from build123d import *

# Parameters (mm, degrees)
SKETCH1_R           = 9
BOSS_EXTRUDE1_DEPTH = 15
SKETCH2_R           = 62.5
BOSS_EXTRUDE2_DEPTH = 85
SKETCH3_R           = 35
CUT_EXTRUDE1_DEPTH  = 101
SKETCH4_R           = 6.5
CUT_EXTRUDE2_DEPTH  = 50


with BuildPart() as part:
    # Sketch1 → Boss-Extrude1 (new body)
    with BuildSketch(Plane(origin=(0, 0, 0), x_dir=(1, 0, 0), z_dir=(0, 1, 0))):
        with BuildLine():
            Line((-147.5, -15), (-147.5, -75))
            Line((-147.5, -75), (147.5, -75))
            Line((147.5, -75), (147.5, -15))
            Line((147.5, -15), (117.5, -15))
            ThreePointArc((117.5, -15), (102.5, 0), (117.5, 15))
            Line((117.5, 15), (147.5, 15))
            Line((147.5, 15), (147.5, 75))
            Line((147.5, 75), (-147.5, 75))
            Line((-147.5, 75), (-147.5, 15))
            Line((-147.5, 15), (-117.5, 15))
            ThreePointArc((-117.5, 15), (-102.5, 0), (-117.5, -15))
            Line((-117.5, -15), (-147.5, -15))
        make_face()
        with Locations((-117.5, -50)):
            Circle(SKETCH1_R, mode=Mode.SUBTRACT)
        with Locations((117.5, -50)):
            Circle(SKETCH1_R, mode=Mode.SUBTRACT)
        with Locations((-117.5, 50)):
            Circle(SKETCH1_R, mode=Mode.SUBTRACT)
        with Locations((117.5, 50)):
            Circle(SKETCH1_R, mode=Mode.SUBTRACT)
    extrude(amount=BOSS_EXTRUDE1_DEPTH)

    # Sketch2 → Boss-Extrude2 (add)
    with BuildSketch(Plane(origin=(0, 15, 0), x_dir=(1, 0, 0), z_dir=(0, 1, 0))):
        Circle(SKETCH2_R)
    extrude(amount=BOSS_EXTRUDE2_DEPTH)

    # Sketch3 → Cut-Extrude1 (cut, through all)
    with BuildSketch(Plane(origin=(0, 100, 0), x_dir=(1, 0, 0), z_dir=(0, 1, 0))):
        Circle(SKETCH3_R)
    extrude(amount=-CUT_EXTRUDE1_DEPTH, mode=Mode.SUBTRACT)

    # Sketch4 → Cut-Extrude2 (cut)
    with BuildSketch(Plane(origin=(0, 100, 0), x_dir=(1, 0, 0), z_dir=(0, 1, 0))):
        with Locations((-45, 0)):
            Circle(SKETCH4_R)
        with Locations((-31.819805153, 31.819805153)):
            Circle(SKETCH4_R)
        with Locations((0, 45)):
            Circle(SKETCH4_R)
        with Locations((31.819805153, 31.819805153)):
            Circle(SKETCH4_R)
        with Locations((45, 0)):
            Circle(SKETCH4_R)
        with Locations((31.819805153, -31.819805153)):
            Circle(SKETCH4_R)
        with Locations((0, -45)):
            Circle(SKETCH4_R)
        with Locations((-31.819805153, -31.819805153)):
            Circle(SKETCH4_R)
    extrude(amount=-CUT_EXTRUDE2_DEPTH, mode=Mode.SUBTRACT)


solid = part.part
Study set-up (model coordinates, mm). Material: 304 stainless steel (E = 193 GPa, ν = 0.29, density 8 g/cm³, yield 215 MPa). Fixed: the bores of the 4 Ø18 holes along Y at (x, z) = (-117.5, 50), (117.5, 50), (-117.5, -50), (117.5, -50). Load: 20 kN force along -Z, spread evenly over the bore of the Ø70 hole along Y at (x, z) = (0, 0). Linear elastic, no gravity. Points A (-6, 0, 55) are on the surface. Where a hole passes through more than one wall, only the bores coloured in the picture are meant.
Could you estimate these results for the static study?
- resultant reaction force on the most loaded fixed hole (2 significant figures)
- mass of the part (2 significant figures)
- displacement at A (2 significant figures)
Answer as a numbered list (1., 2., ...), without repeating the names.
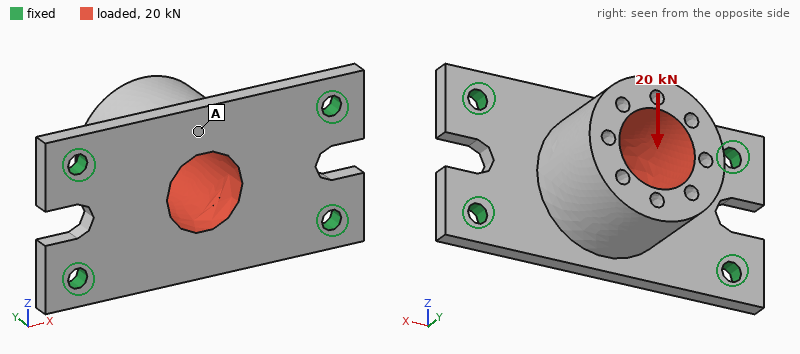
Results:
1. 8.1 kN
2. 9.7 kg
3. 0.047 mm
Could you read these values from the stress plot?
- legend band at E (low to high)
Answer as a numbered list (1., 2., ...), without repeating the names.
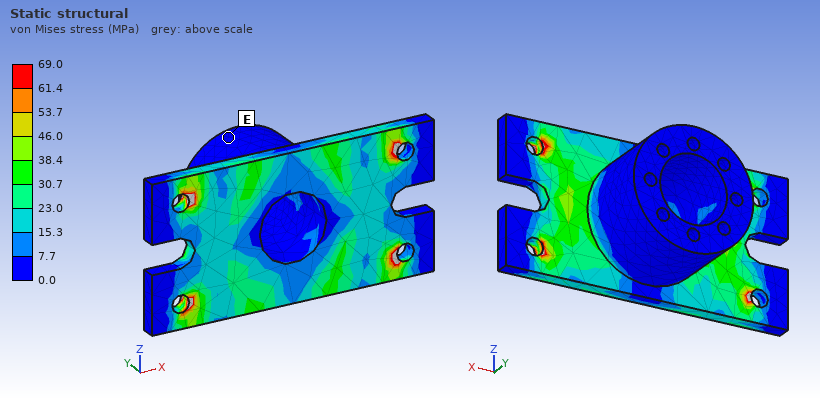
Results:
1. 0.0 to 7.7 MPa
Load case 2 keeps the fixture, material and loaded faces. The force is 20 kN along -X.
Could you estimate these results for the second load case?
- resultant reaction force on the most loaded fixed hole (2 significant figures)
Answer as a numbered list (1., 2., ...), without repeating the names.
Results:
1. 5.7 kN
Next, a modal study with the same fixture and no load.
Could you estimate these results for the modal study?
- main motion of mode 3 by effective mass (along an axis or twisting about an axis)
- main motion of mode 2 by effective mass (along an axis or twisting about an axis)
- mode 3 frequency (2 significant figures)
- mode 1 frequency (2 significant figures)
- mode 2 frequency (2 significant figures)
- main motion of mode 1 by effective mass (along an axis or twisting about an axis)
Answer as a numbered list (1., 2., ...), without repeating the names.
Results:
1. along X
2. along Y
3. 1700 Hz
4. 950 Hz
5. 1200 Hz
6. along Z
